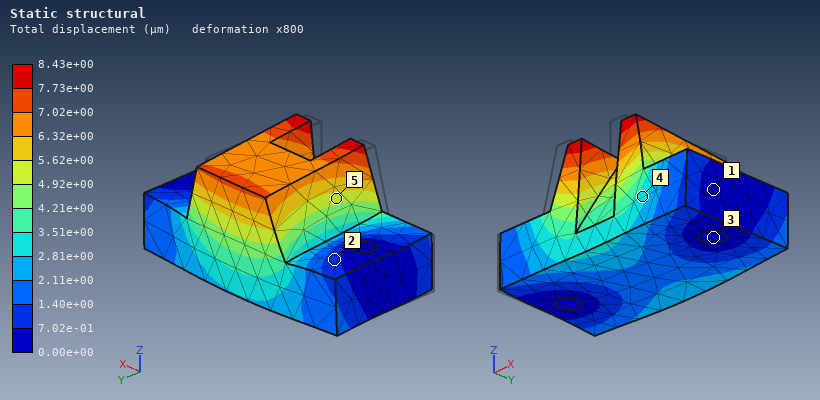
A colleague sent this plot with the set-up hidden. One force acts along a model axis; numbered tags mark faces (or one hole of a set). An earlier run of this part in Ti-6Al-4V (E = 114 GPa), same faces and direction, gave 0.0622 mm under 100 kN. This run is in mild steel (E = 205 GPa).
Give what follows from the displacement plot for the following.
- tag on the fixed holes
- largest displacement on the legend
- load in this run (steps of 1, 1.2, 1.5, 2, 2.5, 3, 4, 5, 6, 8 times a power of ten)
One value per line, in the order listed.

3
8.43e+00 µm
25 kN
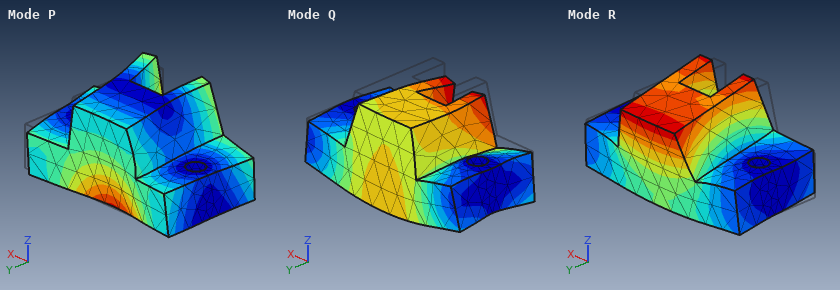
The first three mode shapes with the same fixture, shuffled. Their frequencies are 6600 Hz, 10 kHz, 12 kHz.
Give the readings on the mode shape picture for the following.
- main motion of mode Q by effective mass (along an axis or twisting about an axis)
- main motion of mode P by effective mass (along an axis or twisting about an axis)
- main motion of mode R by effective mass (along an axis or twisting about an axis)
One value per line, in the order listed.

along Z
along Y
along Y
